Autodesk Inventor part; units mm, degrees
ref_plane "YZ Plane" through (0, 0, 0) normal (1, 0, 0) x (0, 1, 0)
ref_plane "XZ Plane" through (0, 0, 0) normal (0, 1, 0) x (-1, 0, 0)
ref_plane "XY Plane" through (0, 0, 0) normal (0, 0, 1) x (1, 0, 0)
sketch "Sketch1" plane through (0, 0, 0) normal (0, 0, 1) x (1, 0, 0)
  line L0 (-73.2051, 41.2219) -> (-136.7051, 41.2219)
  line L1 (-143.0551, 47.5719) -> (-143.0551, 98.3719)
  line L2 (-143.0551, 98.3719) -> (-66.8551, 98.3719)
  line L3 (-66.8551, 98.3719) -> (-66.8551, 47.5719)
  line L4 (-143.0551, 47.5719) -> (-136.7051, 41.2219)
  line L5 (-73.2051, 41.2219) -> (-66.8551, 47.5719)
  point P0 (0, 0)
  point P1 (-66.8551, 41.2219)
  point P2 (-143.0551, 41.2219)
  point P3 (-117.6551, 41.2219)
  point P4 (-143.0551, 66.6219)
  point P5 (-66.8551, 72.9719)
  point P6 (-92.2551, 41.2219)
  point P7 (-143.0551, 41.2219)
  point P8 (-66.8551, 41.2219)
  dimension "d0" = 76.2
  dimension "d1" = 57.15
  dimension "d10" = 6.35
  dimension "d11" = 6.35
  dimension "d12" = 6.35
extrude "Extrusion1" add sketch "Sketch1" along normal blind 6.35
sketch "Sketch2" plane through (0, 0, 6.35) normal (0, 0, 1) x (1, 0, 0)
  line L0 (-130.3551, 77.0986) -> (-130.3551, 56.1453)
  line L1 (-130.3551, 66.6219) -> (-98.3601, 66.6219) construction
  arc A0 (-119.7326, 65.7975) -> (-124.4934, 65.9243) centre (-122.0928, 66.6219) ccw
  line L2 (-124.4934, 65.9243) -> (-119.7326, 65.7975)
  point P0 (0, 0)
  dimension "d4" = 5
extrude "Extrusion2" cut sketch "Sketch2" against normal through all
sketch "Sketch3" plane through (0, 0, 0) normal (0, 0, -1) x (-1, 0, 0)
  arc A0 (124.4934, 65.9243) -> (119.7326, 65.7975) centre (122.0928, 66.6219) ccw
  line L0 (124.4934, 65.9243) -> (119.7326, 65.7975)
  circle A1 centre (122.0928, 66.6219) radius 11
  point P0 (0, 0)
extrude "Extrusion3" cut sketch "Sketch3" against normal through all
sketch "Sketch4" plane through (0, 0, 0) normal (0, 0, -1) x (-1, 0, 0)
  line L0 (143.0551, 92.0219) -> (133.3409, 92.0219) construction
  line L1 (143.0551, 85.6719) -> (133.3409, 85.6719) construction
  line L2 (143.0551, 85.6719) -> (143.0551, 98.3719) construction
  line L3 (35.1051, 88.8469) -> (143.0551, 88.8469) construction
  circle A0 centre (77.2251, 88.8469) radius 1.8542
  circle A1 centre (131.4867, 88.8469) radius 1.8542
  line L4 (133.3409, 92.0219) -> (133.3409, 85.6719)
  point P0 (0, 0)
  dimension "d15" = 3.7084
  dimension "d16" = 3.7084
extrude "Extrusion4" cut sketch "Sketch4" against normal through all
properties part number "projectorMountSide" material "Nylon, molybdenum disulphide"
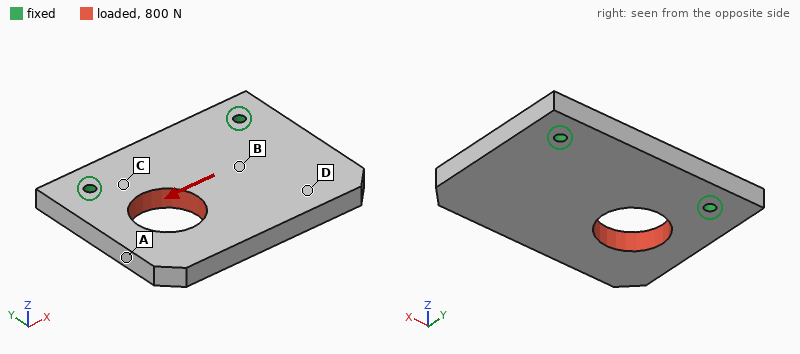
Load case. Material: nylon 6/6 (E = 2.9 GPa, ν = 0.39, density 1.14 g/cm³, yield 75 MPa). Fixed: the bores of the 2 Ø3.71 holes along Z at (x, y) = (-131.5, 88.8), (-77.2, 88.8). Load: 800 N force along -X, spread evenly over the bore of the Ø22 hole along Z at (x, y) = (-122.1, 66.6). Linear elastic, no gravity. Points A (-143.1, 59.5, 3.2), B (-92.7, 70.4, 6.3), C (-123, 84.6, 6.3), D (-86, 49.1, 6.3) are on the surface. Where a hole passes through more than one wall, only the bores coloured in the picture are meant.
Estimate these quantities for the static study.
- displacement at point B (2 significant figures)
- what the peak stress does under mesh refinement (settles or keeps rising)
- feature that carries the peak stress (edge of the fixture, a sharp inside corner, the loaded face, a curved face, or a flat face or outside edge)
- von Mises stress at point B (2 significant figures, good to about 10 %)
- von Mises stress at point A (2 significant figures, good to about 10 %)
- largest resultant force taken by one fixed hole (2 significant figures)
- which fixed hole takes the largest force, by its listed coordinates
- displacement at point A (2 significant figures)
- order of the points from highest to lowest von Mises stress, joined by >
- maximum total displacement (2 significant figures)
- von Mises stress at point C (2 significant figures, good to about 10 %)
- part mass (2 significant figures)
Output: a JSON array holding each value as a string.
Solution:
["0.050 mm", "keeps rising", "edge of the fixture", "2.9 MPa", "5.0 MPa", "560 N", "(-131.5, 88.8)", "0.13 mm", "C > A > B > D", "0.13 mm", "7.1 MPa", "28 g"]
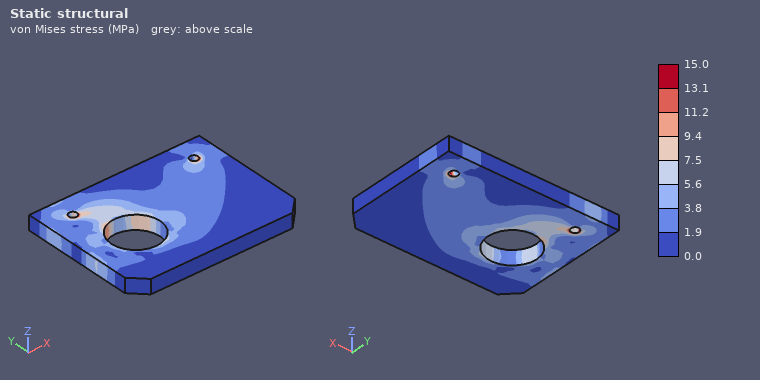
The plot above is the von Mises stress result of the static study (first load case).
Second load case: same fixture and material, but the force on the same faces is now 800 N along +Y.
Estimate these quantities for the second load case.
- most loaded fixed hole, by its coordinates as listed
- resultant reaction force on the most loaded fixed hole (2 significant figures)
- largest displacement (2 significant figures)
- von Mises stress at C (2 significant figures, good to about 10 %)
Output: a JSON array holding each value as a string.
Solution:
["(-131.5, 88.8)", "660 N", "88 µm", "4.6 MPa"]
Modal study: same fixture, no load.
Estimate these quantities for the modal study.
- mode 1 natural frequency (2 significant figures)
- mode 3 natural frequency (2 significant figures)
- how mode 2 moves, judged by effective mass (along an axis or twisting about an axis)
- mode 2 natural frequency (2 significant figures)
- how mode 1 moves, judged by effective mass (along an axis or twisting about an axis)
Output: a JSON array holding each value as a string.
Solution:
["570 Hz", "2300 Hz", "twisting about Y", "1200 Hz", "along Z"]
